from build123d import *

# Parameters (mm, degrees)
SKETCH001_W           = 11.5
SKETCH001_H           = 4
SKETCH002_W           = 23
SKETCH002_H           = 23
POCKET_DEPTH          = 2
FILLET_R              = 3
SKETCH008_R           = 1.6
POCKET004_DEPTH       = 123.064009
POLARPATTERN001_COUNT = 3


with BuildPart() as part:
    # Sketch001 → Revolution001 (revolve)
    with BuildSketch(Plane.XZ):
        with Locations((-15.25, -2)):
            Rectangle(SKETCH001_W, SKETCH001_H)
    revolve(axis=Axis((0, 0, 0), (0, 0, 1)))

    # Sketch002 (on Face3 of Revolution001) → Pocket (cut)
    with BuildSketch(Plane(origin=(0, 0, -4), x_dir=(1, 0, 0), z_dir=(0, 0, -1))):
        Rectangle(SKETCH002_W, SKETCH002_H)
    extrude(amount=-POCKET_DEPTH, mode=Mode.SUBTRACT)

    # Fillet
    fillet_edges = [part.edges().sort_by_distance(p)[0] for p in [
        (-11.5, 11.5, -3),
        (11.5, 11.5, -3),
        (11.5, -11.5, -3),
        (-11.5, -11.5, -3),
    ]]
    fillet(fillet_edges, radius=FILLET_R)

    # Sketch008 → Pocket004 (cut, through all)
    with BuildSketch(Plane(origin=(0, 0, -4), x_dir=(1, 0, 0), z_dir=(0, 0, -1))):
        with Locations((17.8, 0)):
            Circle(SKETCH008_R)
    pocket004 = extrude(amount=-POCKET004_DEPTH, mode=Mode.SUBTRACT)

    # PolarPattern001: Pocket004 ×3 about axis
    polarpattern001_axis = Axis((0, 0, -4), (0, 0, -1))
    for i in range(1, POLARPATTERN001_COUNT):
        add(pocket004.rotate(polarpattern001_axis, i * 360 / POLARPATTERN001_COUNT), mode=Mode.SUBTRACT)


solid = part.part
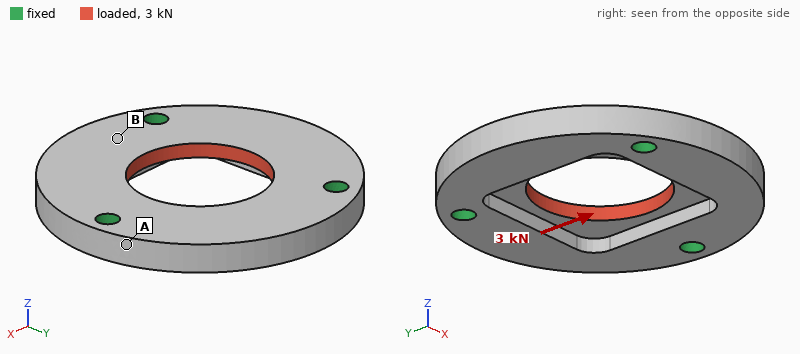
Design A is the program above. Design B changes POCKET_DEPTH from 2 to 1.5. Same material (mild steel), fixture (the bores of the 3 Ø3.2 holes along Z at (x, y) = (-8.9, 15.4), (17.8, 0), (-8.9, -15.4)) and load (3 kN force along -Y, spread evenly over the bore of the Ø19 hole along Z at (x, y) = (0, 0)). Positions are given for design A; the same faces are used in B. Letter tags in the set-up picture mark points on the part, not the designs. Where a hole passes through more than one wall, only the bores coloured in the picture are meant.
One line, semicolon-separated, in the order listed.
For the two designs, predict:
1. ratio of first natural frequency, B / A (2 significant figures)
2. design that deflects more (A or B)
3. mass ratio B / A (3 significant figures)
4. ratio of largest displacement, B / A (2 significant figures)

1.0; A; 1.03; 0.83
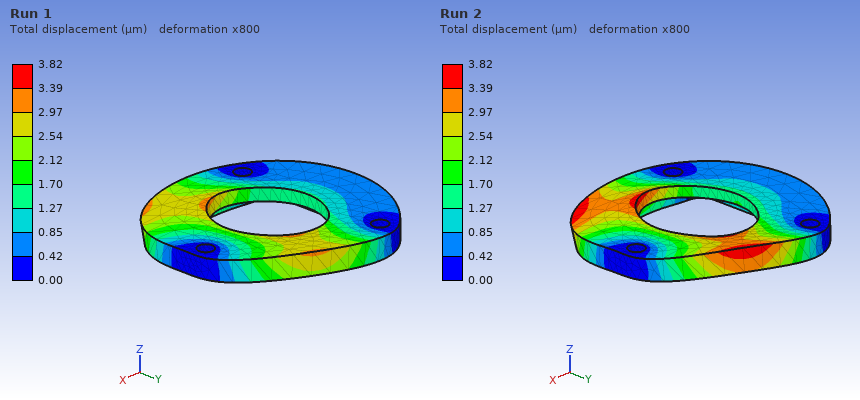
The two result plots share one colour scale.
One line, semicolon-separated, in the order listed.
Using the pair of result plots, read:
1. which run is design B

Run 1
